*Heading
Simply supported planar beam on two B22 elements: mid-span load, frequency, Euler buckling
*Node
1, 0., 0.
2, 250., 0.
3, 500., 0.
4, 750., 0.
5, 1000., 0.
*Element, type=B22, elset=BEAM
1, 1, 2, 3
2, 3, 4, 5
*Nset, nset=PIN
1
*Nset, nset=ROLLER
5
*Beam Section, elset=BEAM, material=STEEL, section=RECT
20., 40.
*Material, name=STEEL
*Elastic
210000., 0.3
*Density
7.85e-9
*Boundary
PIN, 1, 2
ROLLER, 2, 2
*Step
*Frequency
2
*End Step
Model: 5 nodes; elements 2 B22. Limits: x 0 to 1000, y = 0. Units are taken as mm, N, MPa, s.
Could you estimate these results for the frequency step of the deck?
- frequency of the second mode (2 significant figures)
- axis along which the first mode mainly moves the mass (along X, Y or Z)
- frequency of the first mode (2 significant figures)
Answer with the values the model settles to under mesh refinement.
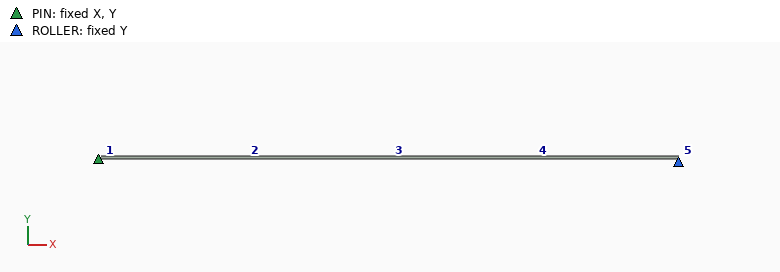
370 Hz
along Y
94 Hz
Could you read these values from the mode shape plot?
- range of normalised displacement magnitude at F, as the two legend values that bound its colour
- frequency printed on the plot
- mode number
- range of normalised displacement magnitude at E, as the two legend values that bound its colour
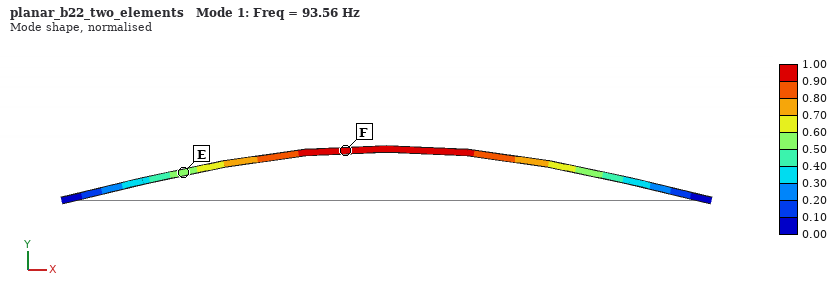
0.90 to 1.00
93.56 Hz
1
0.50 to 0.60
